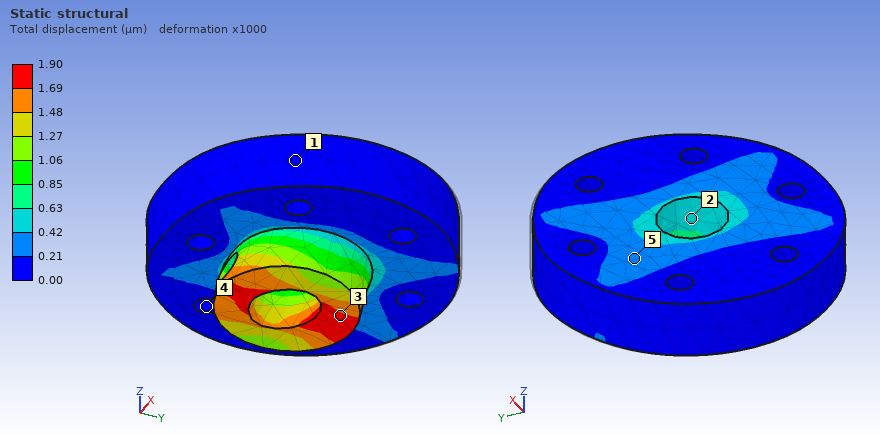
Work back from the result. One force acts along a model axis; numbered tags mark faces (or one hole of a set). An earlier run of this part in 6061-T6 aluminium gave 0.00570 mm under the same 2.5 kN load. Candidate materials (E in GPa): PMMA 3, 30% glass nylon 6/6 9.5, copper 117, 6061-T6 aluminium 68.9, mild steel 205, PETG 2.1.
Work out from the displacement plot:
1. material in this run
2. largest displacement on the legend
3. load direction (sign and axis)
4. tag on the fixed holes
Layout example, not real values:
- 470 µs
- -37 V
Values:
- mild steel
- 1.90 µm
- -Y
- 4
